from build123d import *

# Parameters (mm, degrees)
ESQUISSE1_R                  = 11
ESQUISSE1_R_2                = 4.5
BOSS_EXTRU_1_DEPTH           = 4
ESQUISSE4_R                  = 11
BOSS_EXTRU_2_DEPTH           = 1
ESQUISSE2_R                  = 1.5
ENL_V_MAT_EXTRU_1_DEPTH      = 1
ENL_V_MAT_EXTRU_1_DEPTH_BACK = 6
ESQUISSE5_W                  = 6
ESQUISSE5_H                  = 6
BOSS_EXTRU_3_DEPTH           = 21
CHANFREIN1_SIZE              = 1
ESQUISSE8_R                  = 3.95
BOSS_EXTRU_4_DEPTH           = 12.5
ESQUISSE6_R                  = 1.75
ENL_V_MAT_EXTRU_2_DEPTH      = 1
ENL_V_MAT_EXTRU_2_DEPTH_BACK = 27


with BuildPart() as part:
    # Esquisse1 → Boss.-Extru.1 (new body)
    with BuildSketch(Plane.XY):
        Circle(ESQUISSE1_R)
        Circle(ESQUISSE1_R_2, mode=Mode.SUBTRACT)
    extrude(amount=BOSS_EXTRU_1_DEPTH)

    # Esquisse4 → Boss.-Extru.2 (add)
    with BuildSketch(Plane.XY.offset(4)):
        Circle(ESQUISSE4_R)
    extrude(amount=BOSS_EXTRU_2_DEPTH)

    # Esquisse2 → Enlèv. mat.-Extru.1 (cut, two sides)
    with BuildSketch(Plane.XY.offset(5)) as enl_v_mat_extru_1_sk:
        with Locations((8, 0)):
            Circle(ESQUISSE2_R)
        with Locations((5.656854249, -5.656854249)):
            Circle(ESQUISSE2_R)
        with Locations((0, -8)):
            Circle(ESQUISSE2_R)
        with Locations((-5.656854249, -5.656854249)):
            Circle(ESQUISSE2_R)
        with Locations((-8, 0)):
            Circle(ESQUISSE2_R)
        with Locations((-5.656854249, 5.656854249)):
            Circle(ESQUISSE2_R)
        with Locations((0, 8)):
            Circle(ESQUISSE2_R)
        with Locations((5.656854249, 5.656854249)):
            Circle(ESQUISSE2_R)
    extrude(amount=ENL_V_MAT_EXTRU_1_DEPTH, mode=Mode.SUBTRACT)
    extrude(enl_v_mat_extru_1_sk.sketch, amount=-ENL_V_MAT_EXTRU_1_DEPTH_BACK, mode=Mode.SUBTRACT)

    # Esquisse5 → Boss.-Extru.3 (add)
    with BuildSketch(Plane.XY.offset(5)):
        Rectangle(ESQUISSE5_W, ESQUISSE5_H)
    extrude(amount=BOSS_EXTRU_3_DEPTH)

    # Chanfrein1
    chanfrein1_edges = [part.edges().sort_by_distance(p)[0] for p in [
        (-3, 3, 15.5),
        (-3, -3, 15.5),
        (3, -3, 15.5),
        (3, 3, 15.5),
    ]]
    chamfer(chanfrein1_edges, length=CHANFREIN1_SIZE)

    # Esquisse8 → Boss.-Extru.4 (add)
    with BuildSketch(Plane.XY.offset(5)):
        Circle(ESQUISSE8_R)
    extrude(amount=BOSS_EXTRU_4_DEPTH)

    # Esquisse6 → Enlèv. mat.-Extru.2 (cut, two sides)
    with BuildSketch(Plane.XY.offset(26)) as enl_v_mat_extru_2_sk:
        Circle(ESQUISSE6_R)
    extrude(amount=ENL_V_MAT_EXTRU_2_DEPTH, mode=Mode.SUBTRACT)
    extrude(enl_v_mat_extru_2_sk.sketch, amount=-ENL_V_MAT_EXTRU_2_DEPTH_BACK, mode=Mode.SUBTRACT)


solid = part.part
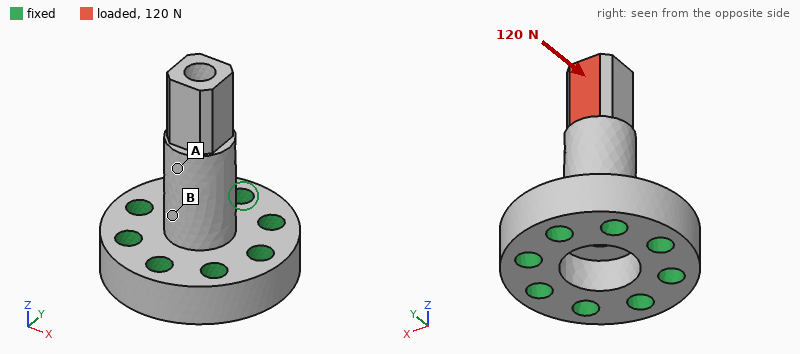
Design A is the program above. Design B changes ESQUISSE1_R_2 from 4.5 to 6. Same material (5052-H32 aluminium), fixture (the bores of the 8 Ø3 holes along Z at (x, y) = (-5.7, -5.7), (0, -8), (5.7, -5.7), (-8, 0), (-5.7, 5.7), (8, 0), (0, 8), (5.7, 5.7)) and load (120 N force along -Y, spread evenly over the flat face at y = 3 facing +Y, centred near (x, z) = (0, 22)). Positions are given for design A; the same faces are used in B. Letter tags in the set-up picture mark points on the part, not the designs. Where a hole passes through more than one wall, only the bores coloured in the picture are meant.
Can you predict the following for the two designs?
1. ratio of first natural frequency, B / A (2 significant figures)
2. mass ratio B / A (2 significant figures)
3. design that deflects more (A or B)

0.75
0.90
B
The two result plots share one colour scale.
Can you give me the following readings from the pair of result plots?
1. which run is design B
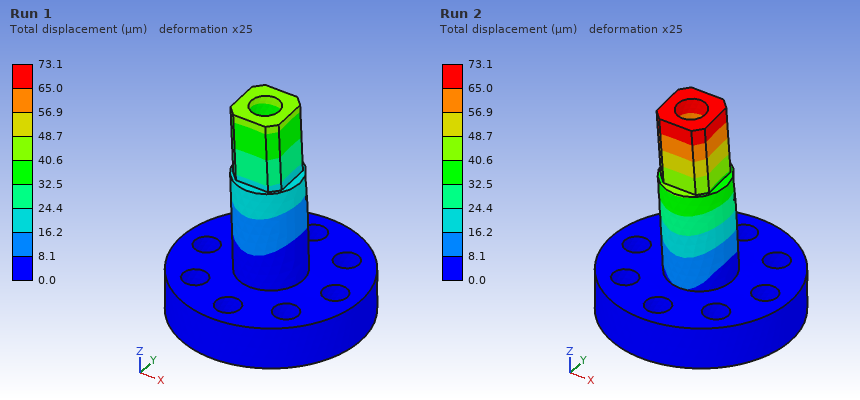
Run 2
